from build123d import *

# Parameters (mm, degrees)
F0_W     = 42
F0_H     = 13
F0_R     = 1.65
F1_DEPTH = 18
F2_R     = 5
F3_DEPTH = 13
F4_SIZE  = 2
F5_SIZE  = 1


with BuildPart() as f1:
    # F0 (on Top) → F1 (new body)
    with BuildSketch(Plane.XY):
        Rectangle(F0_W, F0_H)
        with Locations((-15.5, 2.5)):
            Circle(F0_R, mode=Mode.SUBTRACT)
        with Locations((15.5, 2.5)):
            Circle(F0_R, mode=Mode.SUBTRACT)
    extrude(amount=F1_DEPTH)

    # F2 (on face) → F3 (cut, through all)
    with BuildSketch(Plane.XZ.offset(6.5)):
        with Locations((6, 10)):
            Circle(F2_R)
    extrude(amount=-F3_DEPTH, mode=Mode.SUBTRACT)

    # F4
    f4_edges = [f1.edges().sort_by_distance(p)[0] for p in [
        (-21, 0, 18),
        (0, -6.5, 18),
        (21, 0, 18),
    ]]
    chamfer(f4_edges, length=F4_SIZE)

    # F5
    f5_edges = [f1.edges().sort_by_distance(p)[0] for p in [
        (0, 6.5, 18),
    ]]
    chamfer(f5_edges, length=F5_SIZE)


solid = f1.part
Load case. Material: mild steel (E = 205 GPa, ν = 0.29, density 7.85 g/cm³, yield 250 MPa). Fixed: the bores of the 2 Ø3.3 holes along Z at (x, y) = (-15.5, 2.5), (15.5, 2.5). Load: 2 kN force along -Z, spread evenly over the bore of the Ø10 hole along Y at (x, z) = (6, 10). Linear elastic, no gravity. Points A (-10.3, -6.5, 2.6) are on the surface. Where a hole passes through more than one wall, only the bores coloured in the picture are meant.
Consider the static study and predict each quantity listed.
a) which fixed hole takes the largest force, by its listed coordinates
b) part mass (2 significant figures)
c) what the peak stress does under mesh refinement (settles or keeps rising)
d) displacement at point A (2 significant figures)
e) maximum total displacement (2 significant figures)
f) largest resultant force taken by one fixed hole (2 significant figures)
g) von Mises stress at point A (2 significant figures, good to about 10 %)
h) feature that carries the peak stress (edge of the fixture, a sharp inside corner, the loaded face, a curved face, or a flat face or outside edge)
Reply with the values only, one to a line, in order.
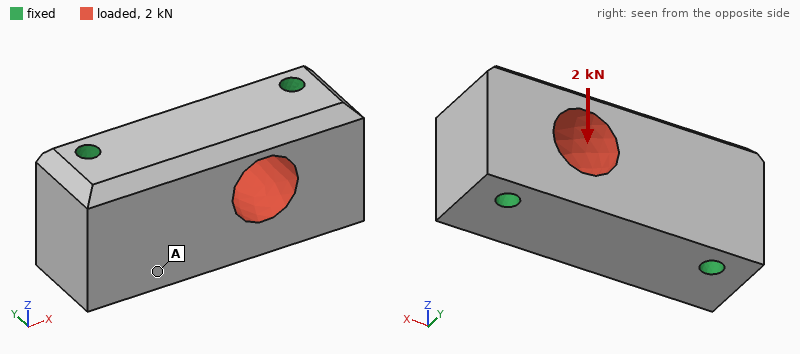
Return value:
(15.5, 2.5)
66 g
keeps rising
0.52 µm
1.8 µm
1.3 kN
3.4 MPa
edge of the fixture
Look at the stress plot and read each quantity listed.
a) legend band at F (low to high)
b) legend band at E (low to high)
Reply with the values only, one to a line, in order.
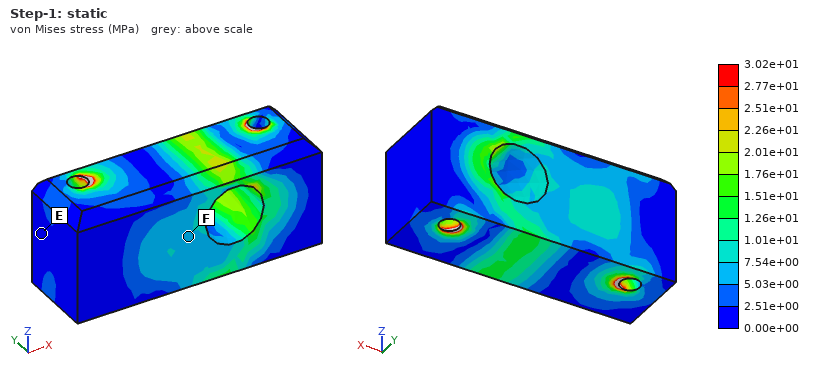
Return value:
5.03e+00 to 7.54e+00 MPa
0.00e+00 to 2.51e+00 MPa
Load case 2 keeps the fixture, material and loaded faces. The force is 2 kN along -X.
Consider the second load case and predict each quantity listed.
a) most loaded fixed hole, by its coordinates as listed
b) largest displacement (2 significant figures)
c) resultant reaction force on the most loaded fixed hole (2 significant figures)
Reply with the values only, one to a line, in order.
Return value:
(15.5, 2.5)
0.56 µm
1.2 kN
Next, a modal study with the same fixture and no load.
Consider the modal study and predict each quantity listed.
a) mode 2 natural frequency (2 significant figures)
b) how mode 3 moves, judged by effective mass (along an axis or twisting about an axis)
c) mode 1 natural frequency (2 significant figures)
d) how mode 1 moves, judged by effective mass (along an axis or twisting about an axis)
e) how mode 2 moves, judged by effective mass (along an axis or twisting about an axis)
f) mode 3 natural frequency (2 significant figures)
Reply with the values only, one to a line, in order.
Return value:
36 kHz
twisting about X
31 kHz
along Y
along Z
43 kHz
